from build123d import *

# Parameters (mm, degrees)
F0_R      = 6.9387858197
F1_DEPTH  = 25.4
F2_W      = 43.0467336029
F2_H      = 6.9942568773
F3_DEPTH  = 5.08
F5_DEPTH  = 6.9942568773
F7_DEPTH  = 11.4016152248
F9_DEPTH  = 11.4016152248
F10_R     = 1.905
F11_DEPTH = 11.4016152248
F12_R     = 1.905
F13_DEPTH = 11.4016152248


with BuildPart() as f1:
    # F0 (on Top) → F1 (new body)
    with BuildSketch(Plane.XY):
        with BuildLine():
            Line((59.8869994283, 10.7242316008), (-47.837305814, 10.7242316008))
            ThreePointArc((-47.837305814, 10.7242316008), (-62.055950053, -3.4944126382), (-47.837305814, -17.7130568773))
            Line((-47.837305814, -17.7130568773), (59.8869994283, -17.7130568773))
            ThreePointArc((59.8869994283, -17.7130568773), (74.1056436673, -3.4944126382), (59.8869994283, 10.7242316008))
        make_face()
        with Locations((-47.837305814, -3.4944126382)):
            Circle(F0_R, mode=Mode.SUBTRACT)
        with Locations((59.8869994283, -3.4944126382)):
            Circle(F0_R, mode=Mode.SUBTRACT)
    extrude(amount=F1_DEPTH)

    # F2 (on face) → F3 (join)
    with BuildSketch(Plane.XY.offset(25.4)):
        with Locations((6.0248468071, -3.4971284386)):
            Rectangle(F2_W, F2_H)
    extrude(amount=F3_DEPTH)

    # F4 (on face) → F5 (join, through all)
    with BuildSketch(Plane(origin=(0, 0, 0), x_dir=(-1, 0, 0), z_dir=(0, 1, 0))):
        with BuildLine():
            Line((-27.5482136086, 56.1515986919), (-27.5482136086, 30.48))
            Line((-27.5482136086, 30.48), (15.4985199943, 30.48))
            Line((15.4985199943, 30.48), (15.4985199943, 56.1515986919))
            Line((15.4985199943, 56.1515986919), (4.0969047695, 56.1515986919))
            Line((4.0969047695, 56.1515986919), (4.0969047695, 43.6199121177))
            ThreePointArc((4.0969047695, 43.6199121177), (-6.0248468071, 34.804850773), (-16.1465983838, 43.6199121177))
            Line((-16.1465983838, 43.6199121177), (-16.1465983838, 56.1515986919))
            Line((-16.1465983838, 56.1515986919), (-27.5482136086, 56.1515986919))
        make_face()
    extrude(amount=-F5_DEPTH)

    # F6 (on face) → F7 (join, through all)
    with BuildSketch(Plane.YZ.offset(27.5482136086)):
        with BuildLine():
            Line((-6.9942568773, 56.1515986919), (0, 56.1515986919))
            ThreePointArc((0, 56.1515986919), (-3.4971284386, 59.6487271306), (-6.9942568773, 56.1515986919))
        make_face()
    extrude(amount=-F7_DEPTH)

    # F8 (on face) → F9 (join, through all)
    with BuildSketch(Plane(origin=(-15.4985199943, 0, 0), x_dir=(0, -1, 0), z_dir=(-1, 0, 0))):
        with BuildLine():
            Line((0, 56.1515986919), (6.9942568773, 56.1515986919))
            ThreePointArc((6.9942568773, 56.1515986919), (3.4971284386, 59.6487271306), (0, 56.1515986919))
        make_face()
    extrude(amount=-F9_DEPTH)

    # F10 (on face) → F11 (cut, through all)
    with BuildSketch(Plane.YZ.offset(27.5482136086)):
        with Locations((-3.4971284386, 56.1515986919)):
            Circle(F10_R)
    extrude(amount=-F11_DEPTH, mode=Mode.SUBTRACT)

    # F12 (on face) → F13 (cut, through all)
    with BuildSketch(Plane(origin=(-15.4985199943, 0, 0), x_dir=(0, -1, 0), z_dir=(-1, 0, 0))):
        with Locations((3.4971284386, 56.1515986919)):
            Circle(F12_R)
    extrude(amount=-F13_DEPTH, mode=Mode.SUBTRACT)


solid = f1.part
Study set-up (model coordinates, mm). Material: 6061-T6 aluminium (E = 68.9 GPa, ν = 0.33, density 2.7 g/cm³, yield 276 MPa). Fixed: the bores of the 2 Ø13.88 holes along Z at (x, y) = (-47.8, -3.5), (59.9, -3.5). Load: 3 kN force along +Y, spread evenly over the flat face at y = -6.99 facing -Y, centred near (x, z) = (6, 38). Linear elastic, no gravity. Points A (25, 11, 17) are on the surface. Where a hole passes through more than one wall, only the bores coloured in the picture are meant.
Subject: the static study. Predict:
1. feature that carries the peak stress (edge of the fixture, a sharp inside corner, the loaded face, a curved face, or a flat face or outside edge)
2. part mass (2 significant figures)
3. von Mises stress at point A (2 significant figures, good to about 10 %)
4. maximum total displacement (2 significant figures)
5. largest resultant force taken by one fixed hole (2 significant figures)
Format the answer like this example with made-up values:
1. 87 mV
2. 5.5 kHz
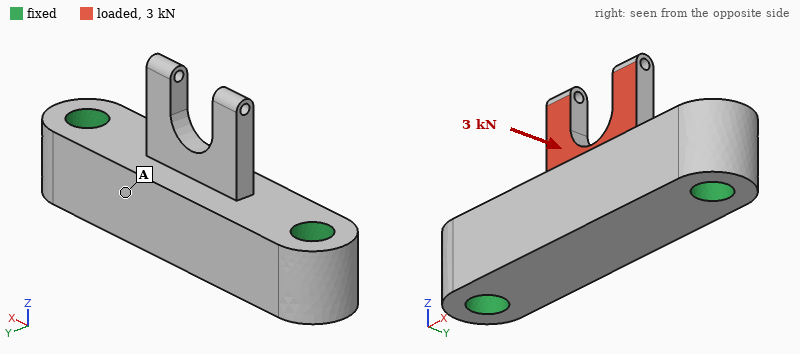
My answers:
1. a flat face or outside edge
2. 250 g
3. 14 MPa
4. 0.23 mm
5. 1.5 kN
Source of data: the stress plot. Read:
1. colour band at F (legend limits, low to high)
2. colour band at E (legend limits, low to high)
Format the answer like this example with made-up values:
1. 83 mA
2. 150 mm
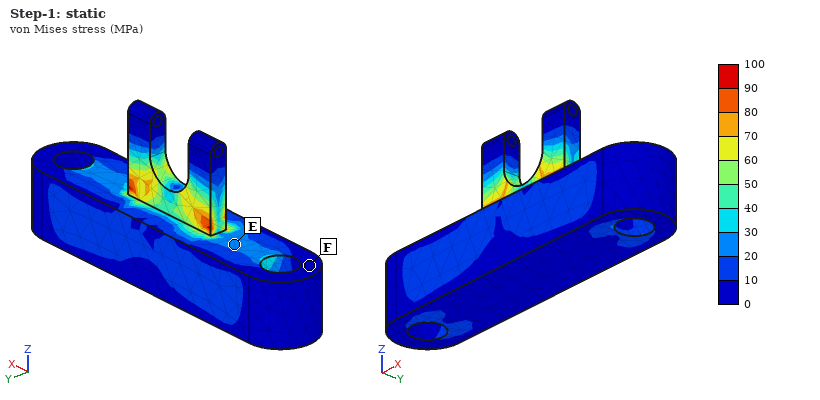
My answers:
1. 0 to 10 MPa
2. 20 to 30 MPa
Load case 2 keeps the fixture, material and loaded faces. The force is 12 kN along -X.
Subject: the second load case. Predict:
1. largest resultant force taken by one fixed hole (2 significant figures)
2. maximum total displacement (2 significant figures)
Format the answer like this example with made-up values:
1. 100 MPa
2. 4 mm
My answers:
1. 7.2 kN
2. 0.20 mm
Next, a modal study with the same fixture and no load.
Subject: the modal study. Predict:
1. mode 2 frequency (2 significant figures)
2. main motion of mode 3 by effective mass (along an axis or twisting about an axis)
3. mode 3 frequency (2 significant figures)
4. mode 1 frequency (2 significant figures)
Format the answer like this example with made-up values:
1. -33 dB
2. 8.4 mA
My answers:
1. 6000 Hz
2. along Y
3. 9100 Hz
4. 5300 Hz
